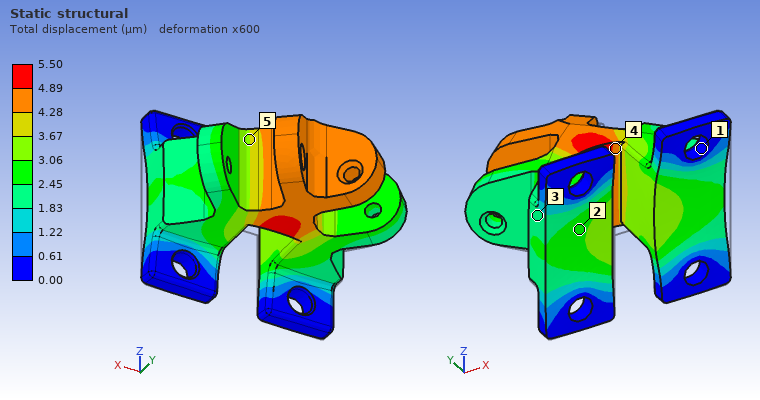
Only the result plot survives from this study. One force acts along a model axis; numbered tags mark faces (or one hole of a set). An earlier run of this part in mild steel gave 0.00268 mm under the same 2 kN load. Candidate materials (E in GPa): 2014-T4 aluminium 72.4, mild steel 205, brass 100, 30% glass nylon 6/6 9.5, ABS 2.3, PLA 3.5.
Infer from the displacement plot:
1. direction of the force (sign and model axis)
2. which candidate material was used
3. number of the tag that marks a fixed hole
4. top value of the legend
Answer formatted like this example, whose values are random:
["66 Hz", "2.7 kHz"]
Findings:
["+Y", "brass", "1", "5.50 µm"]
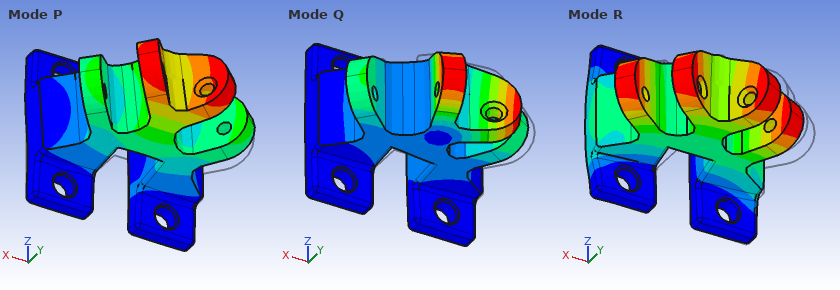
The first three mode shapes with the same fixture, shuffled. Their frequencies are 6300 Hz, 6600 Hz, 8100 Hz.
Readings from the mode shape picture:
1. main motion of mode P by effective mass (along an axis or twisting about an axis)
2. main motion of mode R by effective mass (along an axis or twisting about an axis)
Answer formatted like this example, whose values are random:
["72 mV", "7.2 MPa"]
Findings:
["along Z", "along X"]
